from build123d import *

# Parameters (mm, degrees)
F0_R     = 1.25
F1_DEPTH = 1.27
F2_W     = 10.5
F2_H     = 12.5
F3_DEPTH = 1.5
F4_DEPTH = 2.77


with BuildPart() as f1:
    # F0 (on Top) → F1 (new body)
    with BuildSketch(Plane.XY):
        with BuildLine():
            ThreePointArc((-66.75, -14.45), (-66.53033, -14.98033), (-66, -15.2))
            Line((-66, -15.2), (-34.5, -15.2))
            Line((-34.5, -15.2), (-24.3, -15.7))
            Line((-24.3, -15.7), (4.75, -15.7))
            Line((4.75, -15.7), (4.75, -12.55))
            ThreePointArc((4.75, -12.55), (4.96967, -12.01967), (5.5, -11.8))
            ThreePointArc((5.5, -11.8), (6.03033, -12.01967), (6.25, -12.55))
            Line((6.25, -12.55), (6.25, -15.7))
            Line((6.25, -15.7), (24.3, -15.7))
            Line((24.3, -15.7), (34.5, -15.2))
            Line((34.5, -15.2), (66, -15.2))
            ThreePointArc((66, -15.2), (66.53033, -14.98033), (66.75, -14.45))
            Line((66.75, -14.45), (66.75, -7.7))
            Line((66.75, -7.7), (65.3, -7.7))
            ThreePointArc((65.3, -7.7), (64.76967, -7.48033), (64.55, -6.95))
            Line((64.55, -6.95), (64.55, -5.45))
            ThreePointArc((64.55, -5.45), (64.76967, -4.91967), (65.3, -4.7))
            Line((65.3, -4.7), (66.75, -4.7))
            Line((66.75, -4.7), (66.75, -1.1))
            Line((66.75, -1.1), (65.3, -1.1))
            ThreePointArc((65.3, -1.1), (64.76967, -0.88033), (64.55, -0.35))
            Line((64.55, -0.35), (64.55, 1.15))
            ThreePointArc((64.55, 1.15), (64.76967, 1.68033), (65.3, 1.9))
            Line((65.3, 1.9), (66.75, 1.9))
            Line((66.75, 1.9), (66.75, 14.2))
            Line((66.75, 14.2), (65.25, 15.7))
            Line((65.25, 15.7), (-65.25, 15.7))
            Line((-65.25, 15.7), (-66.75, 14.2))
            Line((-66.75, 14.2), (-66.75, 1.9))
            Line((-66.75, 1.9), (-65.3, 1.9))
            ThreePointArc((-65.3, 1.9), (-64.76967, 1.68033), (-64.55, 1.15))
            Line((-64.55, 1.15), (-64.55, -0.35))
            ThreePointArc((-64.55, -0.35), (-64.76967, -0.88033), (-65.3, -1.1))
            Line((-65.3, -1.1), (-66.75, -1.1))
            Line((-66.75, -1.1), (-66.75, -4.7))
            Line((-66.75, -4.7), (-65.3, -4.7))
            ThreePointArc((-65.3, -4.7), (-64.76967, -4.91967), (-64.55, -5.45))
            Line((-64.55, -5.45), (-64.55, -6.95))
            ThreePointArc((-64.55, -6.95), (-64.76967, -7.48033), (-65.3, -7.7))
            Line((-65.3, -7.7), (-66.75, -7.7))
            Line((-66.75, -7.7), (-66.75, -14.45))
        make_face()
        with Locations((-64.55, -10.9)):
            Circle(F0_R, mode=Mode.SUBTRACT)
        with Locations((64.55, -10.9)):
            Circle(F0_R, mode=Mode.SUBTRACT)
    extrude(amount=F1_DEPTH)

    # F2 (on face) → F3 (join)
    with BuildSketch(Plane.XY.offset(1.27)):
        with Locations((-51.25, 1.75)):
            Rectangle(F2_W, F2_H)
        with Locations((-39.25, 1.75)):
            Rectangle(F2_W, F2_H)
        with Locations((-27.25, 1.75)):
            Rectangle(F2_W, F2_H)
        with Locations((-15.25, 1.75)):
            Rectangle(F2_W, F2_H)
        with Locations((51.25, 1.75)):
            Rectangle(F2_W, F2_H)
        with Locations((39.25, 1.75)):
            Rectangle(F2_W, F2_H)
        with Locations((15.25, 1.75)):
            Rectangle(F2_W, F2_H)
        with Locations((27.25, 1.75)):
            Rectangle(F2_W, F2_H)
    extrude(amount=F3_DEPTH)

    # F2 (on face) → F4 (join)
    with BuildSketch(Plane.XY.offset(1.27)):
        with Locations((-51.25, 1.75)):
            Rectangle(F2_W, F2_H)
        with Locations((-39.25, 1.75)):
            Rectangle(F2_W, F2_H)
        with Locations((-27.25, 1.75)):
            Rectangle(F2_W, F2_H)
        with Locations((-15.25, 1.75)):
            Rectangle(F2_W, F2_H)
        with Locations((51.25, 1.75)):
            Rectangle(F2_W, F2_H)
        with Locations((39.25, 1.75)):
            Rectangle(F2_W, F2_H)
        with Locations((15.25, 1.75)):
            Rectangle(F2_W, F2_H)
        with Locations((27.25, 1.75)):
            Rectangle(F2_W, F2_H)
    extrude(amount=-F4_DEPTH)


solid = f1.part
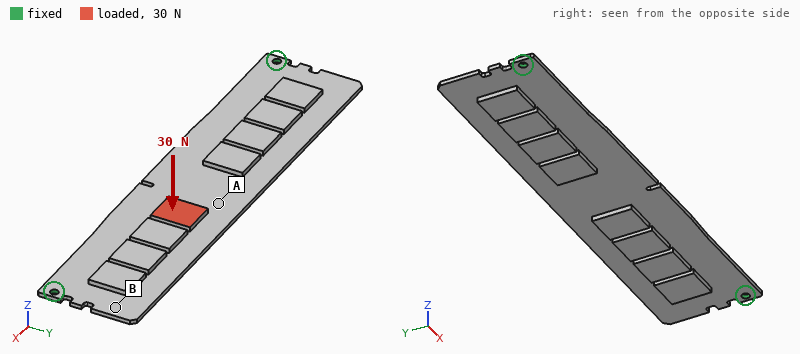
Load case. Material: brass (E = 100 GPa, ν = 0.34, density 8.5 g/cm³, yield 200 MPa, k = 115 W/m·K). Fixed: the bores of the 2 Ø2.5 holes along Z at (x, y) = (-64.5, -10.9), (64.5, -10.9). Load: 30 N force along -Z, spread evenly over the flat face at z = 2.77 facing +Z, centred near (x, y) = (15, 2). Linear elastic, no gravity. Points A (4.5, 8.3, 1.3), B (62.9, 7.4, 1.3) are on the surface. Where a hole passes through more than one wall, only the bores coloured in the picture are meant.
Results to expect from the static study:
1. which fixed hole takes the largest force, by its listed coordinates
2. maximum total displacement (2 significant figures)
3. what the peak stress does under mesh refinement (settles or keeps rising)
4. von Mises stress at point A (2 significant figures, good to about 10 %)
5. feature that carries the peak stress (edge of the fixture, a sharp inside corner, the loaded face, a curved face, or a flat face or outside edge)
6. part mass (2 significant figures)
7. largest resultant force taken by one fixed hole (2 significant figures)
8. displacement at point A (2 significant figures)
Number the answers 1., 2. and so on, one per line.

1. (64.5, -10.9)
2. 0.78 mm
3. keeps rising
4. 53 MPa
5. edge of the fixture
6. 71 g
7. 19 N
8. 0.72 mm
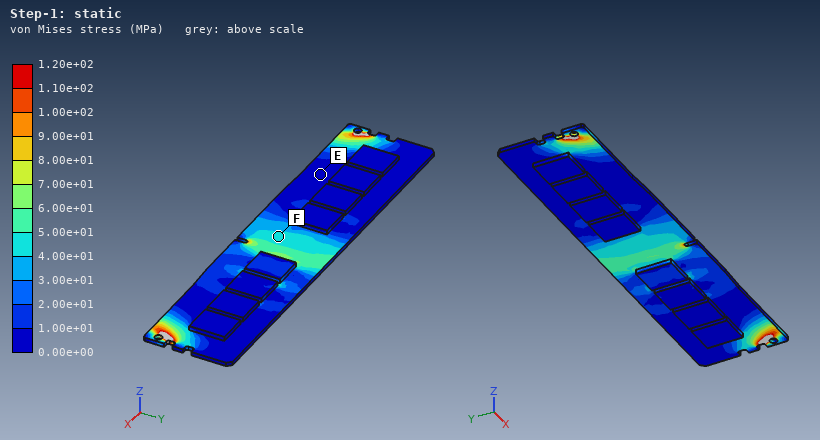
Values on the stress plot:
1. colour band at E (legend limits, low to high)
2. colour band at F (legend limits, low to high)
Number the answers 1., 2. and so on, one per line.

1. 0.00e+00 to 1.00e+01 MPa
2. 4.00e+01 to 5.00e+01 MPa
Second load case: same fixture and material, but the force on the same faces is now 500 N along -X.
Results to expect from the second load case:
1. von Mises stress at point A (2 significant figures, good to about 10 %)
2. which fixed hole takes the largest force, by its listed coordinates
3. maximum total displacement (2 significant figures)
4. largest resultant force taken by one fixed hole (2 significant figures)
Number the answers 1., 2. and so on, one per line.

1. 57 MPa
2. (64.5, -10.9)
3. 0.41 mm
4. 270 N
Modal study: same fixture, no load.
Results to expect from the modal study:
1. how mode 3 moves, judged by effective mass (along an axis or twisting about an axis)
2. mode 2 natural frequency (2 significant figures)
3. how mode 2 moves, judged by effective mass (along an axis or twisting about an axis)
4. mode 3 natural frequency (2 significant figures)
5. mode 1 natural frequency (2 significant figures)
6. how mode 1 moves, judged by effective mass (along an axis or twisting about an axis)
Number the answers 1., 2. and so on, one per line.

1. twisting about Y
2. 550 Hz
3. twisting about X
4. 640 Hz
5. 180 Hz
6. along Z
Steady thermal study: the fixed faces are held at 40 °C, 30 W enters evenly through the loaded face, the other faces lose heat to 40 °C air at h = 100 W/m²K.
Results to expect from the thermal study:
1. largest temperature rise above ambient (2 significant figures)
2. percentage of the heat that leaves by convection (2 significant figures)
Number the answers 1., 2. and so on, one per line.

1. 79 K
2. 86 %
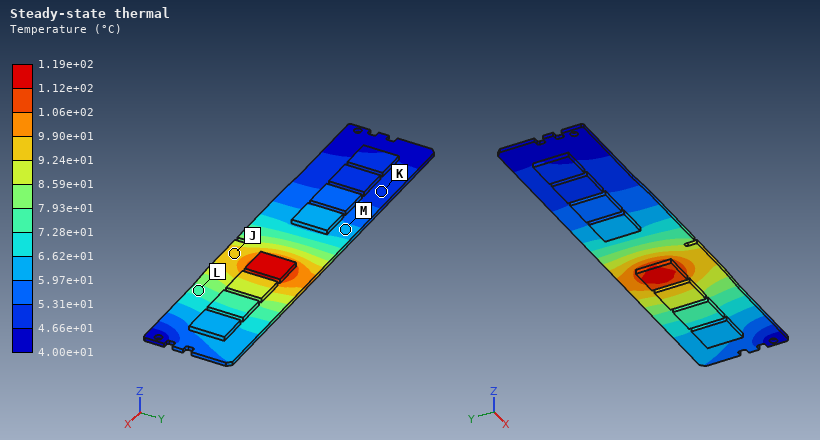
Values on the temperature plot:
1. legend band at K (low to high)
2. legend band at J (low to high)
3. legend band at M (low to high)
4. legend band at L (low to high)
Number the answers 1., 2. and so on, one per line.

1. 4.66e+01 to 5.31e+01 °C
2. 9.24e+01 to 9.90e+01 °C
3. 5.97e+01 to 6.62e+01 °C
4. 7.28e+01 to 7.93e+01 °C
